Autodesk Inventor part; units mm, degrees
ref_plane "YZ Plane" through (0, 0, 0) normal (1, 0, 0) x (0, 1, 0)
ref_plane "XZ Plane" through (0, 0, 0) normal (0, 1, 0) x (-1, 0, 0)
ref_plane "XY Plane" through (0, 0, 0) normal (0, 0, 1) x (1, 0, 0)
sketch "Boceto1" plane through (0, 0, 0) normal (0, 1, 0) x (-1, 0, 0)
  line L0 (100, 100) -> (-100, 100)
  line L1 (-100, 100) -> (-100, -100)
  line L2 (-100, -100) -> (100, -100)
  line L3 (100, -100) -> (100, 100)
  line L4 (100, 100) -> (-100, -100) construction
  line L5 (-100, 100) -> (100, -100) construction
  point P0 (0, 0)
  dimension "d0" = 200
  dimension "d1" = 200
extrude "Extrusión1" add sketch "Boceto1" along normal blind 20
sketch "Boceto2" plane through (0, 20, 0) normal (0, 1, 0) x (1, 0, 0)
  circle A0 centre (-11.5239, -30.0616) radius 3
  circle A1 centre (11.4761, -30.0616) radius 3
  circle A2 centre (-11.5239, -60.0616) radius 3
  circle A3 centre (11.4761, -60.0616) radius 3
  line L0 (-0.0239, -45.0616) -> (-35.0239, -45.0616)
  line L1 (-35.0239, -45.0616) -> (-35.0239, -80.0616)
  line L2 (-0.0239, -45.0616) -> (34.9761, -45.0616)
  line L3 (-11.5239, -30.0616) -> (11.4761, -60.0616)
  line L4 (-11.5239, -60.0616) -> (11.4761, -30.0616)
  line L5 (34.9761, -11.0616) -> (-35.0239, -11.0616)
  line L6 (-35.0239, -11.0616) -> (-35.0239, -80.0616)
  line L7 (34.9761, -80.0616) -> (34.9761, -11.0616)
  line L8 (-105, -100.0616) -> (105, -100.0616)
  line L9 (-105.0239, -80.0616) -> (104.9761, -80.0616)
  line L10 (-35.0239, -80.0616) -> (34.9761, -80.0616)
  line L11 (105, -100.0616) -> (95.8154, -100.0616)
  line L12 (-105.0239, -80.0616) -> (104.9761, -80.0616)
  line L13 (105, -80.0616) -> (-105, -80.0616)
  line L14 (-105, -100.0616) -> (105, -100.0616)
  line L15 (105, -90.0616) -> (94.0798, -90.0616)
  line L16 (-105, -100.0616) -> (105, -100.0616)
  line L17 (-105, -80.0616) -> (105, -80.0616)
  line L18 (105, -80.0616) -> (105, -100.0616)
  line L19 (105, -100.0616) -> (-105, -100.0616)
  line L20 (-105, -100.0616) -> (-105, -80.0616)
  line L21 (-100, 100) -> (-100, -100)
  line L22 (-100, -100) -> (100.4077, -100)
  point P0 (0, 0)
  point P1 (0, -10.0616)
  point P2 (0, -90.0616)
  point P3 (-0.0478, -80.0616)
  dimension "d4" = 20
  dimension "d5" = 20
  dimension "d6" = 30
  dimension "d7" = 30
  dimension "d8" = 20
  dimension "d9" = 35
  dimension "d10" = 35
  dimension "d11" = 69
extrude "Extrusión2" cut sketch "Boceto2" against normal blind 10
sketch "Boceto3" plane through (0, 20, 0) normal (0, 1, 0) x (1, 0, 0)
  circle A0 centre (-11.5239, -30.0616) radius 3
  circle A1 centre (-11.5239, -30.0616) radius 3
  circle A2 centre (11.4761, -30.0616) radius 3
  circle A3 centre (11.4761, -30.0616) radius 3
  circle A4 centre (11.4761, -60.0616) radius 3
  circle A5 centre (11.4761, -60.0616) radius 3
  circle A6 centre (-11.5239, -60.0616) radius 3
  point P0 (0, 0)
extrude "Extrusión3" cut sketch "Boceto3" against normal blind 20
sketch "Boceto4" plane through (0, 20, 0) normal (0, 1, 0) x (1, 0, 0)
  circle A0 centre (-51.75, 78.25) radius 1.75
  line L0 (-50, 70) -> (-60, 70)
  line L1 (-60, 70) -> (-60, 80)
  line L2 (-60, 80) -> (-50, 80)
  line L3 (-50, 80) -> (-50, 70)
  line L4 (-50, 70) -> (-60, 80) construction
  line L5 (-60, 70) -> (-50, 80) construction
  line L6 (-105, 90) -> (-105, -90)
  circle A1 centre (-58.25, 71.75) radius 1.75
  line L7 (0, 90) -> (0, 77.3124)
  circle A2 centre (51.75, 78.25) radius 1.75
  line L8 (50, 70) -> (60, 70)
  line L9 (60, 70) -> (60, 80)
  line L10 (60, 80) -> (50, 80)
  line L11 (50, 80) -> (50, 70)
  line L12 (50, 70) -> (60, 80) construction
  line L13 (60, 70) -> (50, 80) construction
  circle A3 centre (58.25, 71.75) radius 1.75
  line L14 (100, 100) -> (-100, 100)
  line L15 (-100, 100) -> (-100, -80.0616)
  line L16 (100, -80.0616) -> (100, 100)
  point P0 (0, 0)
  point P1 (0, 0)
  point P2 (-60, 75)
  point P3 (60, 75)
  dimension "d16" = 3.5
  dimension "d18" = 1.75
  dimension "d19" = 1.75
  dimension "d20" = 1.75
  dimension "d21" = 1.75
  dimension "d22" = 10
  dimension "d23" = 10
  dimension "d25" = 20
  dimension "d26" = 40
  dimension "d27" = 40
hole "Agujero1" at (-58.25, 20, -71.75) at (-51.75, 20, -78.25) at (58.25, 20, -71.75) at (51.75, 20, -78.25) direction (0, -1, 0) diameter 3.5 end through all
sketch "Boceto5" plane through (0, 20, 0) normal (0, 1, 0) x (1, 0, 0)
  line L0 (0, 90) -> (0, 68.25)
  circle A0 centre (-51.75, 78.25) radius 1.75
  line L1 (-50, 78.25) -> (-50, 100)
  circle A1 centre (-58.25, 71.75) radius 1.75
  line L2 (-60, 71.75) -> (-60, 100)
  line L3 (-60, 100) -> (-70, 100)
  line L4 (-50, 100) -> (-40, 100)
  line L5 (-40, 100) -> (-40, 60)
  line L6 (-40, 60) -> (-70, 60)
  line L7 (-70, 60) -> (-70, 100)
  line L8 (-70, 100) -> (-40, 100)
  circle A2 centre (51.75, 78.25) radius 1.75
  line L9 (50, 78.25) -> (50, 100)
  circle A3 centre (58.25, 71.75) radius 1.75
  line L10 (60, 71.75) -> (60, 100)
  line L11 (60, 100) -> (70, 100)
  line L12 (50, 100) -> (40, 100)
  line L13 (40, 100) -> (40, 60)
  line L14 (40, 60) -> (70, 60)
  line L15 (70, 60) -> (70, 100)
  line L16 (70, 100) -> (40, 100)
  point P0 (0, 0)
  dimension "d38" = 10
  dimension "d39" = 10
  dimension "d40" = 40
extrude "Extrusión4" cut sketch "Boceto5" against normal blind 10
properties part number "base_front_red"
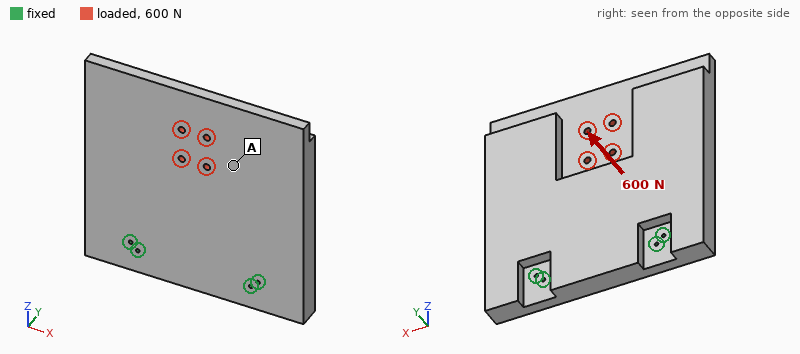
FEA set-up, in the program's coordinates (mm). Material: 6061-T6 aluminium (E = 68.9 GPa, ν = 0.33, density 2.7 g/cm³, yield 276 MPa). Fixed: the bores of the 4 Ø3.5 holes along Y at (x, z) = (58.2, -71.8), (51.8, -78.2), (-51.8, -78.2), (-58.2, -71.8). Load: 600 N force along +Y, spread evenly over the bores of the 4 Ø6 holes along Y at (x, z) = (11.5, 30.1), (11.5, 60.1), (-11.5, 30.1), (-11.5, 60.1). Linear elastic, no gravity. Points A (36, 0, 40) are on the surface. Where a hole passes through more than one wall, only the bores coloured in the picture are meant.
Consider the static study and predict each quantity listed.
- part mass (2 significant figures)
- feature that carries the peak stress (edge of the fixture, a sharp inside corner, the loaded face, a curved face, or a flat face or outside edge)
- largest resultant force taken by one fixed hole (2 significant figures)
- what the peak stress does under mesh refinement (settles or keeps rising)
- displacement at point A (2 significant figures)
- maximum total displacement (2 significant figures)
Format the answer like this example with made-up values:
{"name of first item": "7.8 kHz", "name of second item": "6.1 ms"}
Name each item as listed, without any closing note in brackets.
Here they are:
{"part mass": "1.9 kg", "feature that carries the peak stress": "edge of the fixture", "largest resultant force taken by one fixed hole": "1.3 kN", "what the peak stress does under mesh refinement": "keeps rising", "displacement at point A": "0.15 mm", "maximum total displacement": "0.25 mm"}
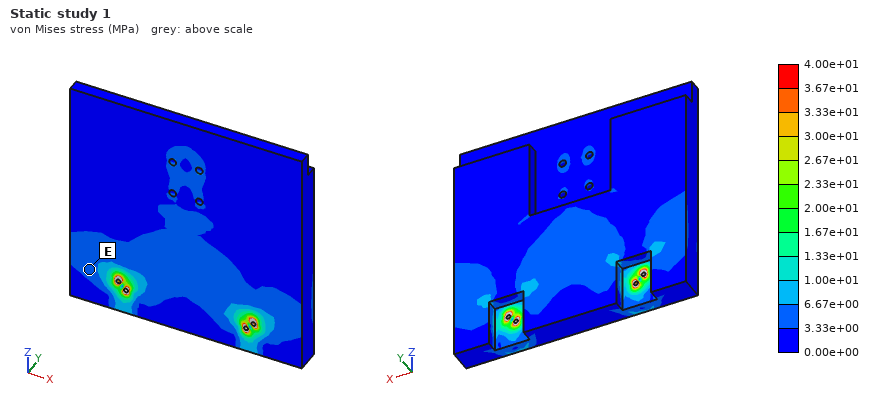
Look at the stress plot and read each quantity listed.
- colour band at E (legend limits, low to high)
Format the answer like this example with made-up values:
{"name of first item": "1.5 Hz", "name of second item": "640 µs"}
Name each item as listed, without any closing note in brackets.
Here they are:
{"colour band at E": "3.33e+00 to 6.67e+00 MPa"}
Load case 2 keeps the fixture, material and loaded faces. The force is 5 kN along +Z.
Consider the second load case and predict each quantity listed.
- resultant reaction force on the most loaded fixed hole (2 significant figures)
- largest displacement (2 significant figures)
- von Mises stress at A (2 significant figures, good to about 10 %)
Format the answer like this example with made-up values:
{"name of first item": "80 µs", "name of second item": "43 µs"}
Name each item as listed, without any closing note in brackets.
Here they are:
{"resultant reaction force on the most loaded fixed hole": "1.4 kN", "largest displacement": "33 µm", "von Mises stress at A": "2.8 MPa"}
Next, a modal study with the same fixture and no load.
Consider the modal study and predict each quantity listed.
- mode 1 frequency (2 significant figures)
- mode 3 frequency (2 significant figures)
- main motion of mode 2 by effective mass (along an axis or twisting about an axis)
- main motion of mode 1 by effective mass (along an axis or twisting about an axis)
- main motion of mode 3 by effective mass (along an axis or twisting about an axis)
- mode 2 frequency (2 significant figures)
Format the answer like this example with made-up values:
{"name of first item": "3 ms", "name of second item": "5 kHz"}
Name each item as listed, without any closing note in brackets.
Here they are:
{"mode 1 frequency": "320 Hz", "mode 3 frequency": "2100 Hz", "main motion of mode 2 by effective mass": "twisting about Z", "main motion of mode 1 by effective mass": "along Y", "main motion of mode 3 by effective mass": "along X", "mode 2 frequency": "840 Hz"}
